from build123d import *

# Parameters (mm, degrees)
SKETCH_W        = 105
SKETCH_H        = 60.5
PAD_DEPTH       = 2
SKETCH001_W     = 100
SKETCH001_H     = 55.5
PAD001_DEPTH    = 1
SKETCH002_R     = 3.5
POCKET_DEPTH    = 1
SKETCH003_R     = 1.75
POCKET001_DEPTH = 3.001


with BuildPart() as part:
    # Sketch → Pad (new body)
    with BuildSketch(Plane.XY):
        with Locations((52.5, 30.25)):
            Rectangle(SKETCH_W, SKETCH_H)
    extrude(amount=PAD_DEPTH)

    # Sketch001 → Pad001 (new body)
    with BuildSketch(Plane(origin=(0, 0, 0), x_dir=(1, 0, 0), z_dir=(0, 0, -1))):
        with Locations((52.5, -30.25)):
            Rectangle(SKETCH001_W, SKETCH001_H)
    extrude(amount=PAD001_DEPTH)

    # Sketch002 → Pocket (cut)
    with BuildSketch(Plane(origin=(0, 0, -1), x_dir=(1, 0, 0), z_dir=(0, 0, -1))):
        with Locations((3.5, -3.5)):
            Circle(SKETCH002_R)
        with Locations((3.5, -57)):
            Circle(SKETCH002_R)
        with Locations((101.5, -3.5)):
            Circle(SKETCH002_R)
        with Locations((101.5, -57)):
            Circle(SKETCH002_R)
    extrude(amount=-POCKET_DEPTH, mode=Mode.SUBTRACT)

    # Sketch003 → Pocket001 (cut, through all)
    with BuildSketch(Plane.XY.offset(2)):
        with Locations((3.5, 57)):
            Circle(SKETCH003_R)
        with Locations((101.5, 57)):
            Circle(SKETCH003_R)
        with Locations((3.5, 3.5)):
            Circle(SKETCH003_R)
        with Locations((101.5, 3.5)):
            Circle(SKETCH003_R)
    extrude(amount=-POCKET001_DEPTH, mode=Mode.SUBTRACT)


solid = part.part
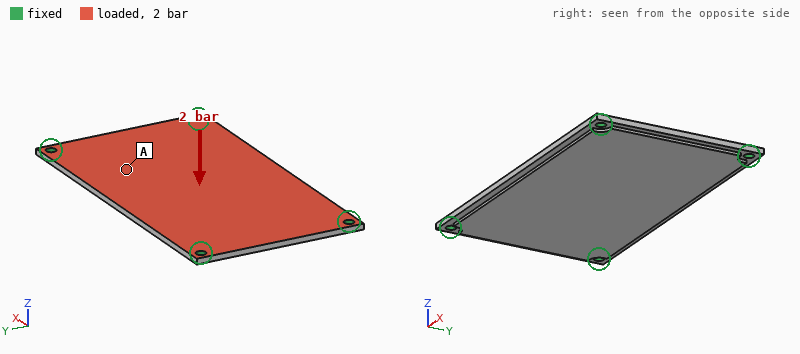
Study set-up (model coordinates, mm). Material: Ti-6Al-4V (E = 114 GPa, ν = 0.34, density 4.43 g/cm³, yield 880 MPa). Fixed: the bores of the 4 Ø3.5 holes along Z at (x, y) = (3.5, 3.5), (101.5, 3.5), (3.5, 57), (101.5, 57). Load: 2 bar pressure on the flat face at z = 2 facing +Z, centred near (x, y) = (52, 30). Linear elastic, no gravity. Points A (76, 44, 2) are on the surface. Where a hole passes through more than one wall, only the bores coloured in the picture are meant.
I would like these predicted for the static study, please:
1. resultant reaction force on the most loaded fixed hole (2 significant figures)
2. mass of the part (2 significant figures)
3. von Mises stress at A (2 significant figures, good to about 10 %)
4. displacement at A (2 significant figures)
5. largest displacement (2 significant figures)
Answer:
640 N
80 g
39 MPa
0.26 mm
0.39 mm
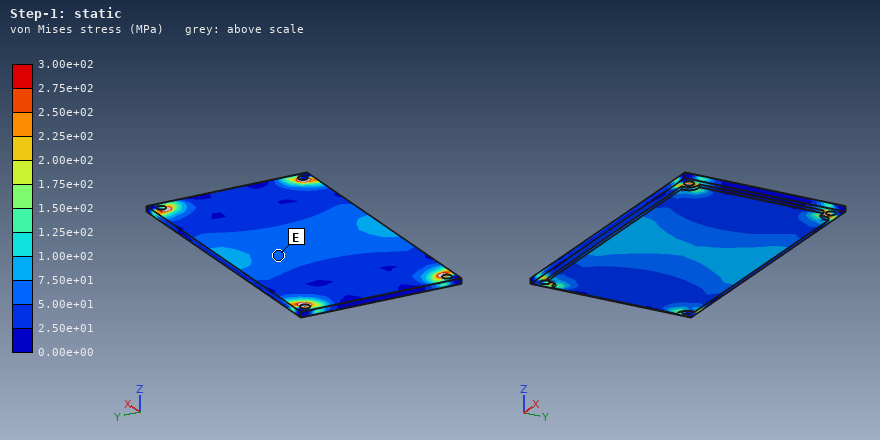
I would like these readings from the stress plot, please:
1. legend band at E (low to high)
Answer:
5.00e+01 to 7.50e+01 MPa
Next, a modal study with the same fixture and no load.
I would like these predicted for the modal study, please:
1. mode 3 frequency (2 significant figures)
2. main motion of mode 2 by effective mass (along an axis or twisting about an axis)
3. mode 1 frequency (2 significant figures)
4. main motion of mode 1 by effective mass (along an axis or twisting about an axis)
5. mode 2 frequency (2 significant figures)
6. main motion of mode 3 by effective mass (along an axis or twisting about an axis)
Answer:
3200 Hz
twisting about X
1200 Hz
along Z
2200 Hz
twisting about Y
